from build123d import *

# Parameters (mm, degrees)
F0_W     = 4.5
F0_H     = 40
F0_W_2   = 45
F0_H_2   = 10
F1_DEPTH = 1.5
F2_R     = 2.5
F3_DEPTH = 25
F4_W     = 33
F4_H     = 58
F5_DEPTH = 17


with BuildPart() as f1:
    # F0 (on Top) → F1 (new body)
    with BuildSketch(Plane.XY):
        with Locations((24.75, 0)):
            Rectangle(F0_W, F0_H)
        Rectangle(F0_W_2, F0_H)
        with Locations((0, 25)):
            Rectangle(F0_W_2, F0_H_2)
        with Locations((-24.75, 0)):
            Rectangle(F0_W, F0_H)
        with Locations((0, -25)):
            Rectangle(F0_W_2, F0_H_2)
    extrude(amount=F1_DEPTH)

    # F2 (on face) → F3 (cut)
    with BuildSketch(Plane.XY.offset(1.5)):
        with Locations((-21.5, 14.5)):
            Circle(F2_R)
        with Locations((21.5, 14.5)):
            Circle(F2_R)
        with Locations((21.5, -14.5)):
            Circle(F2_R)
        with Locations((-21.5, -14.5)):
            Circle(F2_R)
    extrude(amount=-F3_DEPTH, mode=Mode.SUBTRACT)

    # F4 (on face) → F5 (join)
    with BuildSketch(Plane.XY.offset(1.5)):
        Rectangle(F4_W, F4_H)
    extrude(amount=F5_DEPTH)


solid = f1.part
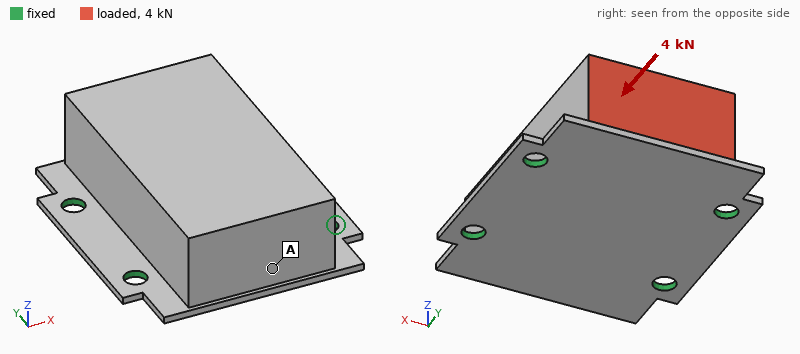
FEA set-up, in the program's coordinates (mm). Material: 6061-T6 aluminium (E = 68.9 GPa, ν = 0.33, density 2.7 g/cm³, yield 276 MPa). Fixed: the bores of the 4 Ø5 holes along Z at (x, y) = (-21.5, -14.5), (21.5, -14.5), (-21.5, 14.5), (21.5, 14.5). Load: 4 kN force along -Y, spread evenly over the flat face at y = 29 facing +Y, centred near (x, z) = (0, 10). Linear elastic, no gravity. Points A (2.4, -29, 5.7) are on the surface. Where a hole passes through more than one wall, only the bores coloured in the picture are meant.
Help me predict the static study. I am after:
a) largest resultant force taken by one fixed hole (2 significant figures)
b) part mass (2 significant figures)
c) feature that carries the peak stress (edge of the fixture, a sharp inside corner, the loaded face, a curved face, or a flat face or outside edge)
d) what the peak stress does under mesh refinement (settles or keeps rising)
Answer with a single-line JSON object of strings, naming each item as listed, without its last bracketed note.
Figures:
{"largest resultant force taken by one fixed hole": "1.3 kN", "part mass": "100 g", "feature that carries the peak stress": "edge of the fixture", "what the peak stress does under mesh refinement": "keeps rising"}
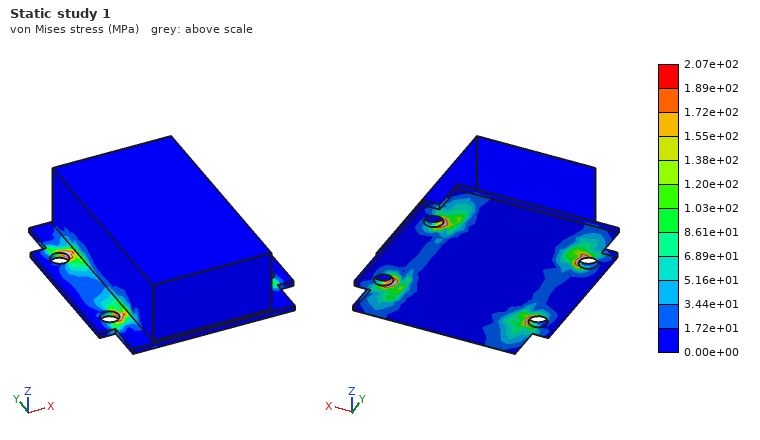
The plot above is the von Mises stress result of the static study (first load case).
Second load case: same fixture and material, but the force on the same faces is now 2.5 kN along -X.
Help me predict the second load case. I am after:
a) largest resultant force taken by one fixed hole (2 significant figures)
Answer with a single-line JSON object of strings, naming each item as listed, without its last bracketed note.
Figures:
{"largest resultant force taken by one fixed hole": "1.3 kN"}
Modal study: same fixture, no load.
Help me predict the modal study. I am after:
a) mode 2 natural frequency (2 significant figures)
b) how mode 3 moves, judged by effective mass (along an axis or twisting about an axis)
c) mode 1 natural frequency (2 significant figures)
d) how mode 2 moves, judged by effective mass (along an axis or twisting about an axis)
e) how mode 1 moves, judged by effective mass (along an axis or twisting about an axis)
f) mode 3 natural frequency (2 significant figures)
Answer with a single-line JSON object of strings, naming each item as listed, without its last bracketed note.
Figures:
{"mode 2 natural frequency": "5600 Hz", "how mode 3 moves, judged by effective mass": "along X", "mode 1 natural frequency": "4100 Hz", "how mode 2 moves, judged by effective mass": "along Z", "how mode 1 moves, judged by effective mass": "along Y", "mode 3 natural frequency": "7200 Hz"}
